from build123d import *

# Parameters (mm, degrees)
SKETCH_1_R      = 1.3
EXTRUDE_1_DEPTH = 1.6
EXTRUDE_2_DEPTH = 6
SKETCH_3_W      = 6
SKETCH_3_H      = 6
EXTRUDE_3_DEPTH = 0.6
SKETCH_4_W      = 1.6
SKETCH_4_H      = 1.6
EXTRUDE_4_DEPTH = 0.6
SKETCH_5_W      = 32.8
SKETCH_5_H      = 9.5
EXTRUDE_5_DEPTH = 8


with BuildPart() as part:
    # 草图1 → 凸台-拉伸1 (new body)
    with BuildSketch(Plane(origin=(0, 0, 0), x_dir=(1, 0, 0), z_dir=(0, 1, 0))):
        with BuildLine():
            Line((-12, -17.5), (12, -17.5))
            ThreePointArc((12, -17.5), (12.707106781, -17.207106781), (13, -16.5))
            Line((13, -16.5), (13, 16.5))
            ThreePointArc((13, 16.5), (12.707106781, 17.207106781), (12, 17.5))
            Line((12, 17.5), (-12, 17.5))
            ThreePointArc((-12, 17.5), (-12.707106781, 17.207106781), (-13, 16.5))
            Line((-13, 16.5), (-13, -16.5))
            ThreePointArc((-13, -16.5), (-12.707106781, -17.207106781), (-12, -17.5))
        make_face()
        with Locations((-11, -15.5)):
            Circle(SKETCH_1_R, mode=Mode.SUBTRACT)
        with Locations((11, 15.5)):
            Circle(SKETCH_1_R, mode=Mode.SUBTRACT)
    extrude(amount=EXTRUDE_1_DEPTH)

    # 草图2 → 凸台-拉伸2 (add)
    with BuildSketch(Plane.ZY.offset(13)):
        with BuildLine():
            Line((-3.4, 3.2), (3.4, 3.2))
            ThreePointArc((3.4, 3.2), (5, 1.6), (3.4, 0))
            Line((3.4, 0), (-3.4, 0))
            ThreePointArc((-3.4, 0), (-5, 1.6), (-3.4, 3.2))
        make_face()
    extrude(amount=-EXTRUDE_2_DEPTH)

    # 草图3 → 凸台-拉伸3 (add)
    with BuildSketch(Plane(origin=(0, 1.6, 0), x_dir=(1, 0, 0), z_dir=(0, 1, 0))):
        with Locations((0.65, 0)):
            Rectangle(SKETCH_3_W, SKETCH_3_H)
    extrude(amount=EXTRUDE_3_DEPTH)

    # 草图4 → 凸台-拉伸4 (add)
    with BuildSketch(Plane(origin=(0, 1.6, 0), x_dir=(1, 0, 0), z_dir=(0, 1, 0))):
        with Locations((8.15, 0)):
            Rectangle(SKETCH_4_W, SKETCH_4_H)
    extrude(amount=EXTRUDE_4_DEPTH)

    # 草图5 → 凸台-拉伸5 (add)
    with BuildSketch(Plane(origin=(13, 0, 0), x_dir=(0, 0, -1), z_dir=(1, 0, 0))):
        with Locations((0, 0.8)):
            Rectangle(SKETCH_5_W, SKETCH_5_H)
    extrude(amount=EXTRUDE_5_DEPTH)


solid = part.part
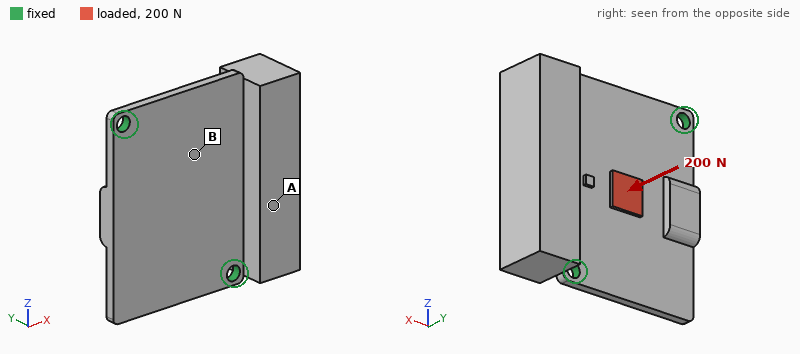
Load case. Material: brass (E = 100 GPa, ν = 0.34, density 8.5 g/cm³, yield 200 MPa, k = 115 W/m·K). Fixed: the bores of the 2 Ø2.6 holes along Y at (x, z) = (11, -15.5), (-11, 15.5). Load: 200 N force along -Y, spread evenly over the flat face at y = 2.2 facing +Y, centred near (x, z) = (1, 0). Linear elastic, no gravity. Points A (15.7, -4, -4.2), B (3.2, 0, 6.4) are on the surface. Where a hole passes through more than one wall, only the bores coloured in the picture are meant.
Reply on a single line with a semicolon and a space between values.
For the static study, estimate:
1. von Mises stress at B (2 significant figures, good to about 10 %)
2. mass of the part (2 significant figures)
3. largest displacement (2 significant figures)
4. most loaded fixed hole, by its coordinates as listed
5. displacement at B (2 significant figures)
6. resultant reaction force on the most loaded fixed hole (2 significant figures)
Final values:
50 MPa; 34 g; 70 µm; (11, -15.5); 53 µm; 110 N
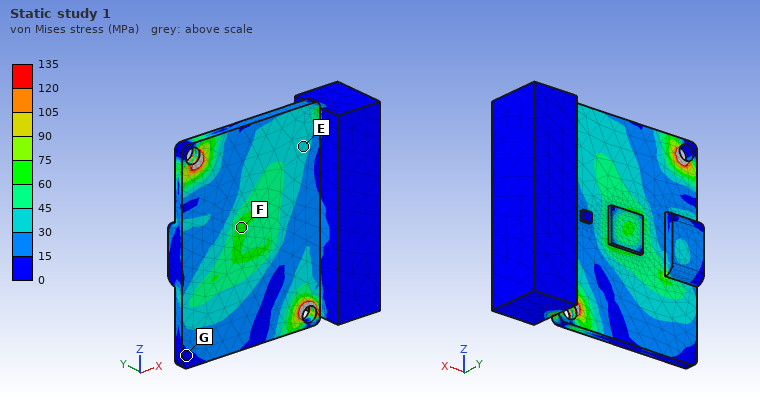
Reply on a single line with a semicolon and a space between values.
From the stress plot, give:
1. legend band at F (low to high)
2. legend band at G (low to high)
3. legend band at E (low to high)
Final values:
60 to 75 MPa; 0 to 15 MPa; 30 to 45 MPa
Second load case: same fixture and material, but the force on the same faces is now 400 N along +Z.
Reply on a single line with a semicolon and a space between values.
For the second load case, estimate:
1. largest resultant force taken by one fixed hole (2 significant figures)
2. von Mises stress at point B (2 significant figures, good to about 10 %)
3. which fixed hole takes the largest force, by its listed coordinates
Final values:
220 N; 15 MPa; (11, -15.5)
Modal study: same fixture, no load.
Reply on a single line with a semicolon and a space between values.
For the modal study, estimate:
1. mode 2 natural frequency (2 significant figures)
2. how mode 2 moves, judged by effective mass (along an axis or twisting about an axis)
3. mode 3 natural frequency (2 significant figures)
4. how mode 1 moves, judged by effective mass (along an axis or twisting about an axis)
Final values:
2400 Hz; along Y; 3900 Hz; along Y
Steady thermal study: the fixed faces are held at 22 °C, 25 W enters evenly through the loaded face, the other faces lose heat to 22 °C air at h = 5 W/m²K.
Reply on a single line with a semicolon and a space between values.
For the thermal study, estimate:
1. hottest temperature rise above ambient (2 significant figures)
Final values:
81 K
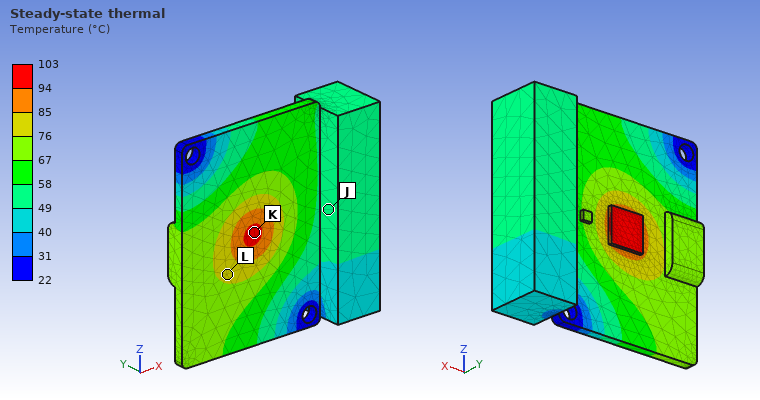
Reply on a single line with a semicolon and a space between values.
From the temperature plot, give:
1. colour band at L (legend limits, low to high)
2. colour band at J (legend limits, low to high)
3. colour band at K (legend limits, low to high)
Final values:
76 to 85 °C; 49 to 58 °C; 94 to 103 °C
